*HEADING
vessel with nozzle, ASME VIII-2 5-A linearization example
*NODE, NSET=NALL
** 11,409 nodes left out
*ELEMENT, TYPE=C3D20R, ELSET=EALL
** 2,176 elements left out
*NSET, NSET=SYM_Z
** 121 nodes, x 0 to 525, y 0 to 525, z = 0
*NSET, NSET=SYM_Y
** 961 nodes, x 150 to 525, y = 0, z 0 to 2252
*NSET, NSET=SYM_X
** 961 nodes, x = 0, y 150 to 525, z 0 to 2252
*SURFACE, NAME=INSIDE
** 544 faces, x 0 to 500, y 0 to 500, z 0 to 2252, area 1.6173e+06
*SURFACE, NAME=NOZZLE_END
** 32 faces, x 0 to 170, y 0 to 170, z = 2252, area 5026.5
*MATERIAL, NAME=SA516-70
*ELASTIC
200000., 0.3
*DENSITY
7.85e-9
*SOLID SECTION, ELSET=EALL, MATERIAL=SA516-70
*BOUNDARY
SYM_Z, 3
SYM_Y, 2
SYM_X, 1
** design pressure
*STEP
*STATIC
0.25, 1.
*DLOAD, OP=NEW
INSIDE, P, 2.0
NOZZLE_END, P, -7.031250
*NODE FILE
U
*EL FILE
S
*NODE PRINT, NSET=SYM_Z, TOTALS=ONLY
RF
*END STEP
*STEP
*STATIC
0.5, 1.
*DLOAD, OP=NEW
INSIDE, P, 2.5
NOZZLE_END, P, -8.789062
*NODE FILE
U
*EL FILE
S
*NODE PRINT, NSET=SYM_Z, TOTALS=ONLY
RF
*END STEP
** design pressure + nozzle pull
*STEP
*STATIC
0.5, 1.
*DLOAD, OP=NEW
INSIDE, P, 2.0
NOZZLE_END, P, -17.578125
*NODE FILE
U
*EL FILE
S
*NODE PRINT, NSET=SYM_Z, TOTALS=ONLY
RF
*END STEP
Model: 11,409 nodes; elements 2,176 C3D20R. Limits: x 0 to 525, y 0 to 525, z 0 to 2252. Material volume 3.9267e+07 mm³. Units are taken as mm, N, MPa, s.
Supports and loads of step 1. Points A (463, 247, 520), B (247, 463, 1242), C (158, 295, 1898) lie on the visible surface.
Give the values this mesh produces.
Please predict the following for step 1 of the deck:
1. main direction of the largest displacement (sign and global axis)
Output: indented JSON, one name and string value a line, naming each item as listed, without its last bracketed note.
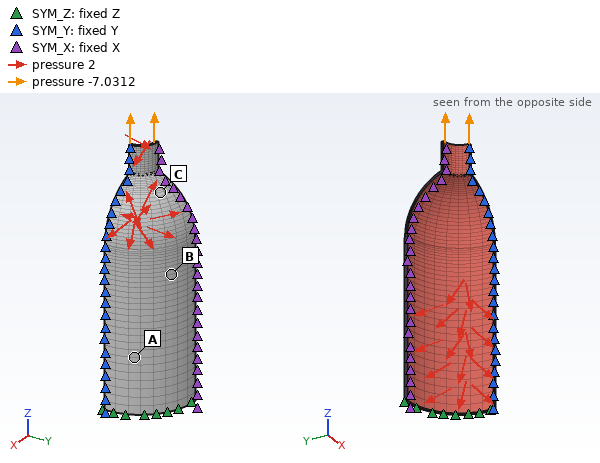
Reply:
{
  "main direction of the largest displacement": "+Z"
}
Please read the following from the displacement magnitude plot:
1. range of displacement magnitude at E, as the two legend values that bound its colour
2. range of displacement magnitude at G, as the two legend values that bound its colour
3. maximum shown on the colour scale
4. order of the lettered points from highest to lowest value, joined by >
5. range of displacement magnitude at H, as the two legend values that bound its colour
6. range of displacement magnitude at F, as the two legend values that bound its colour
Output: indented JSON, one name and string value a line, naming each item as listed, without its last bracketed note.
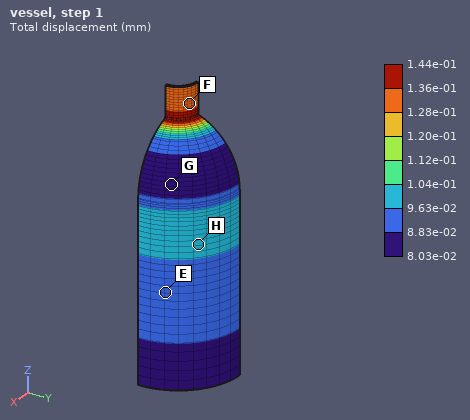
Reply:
{
  "range of displacement magnitude at E, as the two legend values that bound its colour": "8.83e-02 to 9.63e-02 mm",
  "range of displacement magnitude at G, as the two legend values that bound its colour": "8.03e-02 to 8.83e-02 mm",
  "maximum shown on the colour scale": "1.44e-01 mm",
  "order of the lettered points from highest to lowest value, joined by >": "F > H > E > G",
  "range of displacement magnitude at H, as the two legend values that bound its colour": "9.63e-02 to 1.04e-01 mm",
  "range of displacement magnitude at F, as the two legend values that bound its colour": "1.28e-01 to 1.36e-01 mm"
}
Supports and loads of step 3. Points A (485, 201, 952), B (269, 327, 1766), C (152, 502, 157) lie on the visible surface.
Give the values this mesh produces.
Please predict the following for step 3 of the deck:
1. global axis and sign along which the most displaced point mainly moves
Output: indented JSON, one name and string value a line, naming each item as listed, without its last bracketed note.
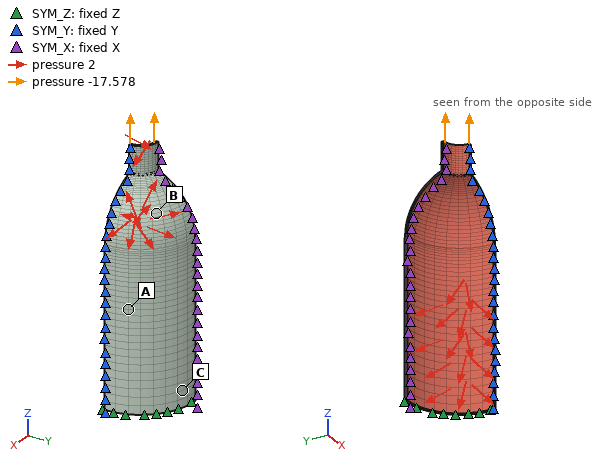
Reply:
{
  "global axis and sign along which the most displaced point mainly moves": "+Z"
}
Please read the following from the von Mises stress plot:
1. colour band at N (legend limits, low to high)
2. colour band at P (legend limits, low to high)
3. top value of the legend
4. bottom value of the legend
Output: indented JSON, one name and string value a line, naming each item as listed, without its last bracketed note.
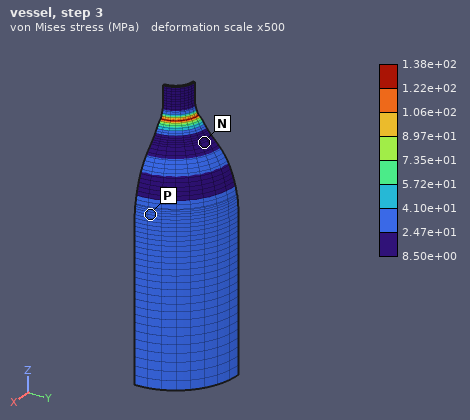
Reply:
{
  "colour band at N": "8.50e+00 to 2.47e+01 MPa",
  "colour band at P": "2.47e+01 to 4.10e+01 MPa",
  "top value of the legend": "1.38e+02 MPa",
  "bottom value of the legend": "8.50e+00 MPa"
}
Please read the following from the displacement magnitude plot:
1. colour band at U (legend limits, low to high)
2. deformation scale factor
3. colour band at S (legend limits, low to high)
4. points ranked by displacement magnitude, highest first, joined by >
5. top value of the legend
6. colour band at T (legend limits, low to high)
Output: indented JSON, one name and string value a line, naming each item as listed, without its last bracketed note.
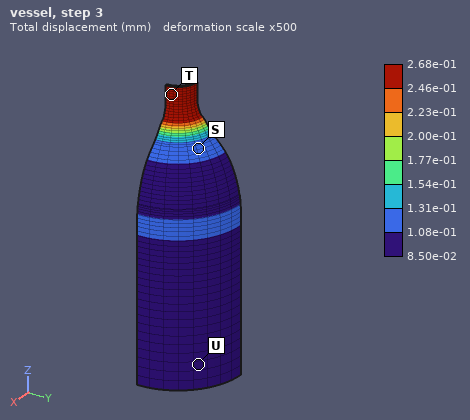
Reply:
{
  "colour band at U": "8.50e-02 to 1.08e-01 mm",
  "deformation scale factor": "500",
  "colour band at S": "1.08e-01 to 1.31e-01 mm",
  "points ranked by displacement magnitude, highest first, joined by >": "T > S > U",
  "top value of the legend": "2.68e-01 mm",
  "colour band at T": "2.46e-01 to 2.68e-01 mm"
}
